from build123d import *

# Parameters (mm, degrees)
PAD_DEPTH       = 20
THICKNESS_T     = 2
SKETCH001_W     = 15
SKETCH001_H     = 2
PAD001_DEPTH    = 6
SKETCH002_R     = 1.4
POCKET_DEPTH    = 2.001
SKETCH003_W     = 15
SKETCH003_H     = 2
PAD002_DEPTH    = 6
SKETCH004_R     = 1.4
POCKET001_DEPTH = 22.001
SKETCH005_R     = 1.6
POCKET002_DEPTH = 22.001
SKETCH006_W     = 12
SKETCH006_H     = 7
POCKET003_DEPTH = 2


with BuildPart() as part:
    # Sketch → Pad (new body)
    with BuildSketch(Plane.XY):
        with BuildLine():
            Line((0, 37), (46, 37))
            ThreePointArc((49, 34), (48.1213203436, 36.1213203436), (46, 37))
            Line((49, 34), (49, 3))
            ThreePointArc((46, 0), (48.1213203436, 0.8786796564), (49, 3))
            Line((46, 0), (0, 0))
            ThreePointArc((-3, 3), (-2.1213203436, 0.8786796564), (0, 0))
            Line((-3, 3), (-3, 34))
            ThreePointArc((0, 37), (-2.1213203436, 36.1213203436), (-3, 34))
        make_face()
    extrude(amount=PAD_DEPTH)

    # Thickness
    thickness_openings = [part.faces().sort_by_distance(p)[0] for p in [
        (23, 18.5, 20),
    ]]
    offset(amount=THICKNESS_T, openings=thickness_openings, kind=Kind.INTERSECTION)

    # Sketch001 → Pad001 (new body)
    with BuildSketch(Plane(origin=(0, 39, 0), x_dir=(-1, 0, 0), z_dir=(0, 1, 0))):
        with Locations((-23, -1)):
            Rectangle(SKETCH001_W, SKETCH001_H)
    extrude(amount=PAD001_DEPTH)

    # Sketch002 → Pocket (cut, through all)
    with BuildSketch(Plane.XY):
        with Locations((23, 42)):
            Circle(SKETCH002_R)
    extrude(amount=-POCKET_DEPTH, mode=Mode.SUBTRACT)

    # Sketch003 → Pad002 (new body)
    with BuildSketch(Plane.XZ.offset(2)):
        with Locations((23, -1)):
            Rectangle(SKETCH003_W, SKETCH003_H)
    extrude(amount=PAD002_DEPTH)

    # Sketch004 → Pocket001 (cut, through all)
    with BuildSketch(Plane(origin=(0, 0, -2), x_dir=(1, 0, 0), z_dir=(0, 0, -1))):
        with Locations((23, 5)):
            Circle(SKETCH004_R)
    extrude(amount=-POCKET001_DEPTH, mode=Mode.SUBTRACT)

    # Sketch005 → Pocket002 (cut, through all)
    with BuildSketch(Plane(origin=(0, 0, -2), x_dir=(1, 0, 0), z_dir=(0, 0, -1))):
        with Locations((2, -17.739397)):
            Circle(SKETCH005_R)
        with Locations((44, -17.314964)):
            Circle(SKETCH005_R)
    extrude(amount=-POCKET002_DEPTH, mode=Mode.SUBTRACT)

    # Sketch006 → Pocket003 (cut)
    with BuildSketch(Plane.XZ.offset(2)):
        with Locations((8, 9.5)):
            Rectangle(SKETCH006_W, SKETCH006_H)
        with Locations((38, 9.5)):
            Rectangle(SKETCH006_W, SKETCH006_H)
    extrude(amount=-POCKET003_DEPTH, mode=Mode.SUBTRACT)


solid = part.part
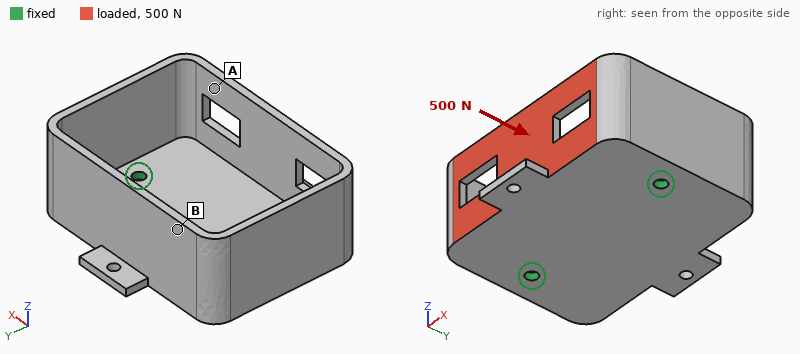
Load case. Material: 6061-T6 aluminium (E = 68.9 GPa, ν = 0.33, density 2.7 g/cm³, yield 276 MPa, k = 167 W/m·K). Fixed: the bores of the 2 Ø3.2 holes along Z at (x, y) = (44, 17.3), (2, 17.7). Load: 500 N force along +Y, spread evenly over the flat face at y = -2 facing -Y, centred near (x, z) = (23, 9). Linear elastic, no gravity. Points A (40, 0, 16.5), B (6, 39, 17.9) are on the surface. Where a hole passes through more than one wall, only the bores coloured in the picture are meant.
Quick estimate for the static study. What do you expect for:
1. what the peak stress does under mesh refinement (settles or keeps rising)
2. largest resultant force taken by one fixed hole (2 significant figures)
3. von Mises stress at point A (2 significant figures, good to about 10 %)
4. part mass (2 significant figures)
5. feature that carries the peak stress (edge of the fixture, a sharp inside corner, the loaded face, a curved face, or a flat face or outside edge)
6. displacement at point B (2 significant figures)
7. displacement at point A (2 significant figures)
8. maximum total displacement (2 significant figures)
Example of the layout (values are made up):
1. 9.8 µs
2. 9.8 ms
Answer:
1. keeps rising
2. 260 N
3. 43 MPa
4. 32 g
5. edge of the fixture
6. 0.17 mm
7. 0.23 mm
8. 0.39 mm
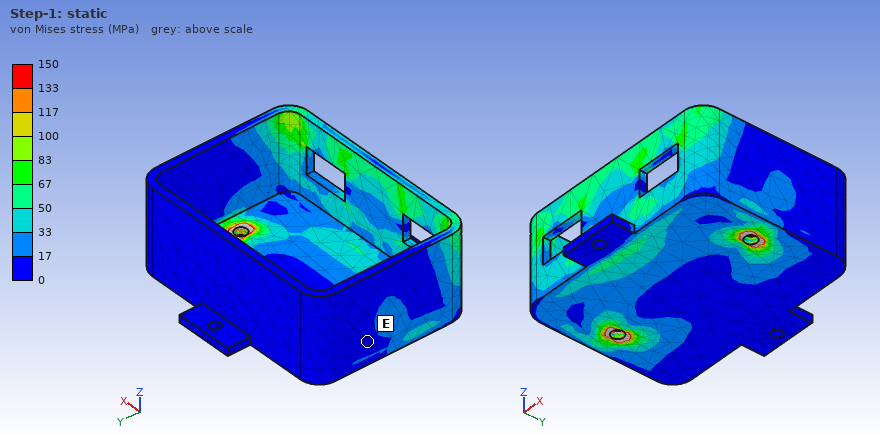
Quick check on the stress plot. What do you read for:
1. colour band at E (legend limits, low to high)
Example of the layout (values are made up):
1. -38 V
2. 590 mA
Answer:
1. 0 to 17 MPa
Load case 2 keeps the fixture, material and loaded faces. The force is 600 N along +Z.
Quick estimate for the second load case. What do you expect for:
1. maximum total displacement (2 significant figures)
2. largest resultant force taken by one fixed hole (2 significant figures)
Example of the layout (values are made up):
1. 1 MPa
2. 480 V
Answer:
1. 0.45 mm
2. 300 N
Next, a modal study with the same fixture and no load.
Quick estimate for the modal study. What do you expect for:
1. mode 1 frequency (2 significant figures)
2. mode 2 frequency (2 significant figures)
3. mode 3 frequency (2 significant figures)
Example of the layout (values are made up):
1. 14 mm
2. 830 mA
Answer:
1. 1500 Hz
2. 2400 Hz
3. 4300 Hz
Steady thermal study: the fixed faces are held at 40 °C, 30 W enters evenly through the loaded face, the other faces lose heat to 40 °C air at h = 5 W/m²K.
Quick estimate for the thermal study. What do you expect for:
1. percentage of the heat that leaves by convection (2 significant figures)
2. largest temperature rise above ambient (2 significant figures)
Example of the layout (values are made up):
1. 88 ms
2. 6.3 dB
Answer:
1. 3.2 %
2. 49 K
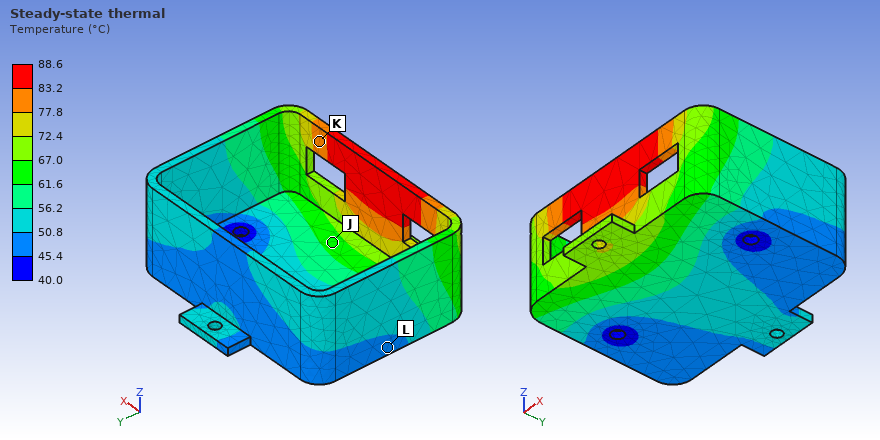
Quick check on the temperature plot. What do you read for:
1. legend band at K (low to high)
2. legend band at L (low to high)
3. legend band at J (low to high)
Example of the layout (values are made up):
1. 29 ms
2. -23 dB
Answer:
1. 77.8 to 83.2 °C
2. 45.4 to 50.8 °C
3. 61.6 to 67.0 °C
